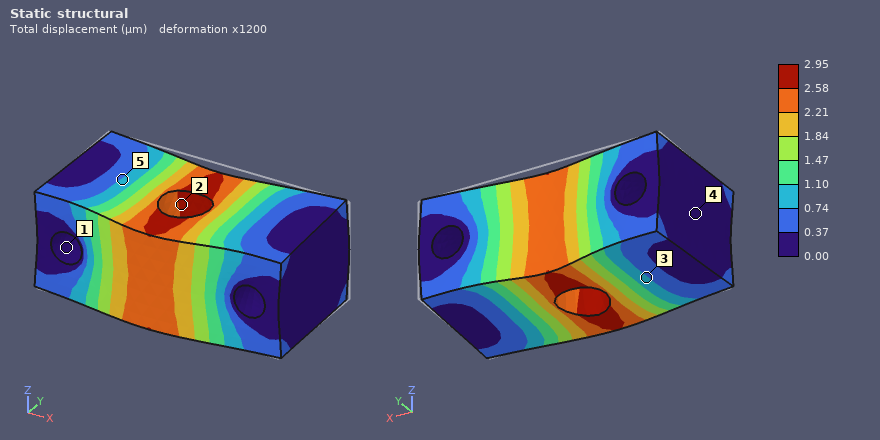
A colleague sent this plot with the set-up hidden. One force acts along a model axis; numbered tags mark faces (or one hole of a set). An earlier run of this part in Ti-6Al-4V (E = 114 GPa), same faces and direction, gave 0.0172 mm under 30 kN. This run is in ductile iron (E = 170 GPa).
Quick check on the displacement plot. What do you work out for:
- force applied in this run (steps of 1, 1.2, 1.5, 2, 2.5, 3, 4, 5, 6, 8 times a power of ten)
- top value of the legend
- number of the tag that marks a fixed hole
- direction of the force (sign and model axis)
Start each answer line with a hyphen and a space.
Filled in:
- 8 kN
- 2.95 µm
- 1
- -Y
